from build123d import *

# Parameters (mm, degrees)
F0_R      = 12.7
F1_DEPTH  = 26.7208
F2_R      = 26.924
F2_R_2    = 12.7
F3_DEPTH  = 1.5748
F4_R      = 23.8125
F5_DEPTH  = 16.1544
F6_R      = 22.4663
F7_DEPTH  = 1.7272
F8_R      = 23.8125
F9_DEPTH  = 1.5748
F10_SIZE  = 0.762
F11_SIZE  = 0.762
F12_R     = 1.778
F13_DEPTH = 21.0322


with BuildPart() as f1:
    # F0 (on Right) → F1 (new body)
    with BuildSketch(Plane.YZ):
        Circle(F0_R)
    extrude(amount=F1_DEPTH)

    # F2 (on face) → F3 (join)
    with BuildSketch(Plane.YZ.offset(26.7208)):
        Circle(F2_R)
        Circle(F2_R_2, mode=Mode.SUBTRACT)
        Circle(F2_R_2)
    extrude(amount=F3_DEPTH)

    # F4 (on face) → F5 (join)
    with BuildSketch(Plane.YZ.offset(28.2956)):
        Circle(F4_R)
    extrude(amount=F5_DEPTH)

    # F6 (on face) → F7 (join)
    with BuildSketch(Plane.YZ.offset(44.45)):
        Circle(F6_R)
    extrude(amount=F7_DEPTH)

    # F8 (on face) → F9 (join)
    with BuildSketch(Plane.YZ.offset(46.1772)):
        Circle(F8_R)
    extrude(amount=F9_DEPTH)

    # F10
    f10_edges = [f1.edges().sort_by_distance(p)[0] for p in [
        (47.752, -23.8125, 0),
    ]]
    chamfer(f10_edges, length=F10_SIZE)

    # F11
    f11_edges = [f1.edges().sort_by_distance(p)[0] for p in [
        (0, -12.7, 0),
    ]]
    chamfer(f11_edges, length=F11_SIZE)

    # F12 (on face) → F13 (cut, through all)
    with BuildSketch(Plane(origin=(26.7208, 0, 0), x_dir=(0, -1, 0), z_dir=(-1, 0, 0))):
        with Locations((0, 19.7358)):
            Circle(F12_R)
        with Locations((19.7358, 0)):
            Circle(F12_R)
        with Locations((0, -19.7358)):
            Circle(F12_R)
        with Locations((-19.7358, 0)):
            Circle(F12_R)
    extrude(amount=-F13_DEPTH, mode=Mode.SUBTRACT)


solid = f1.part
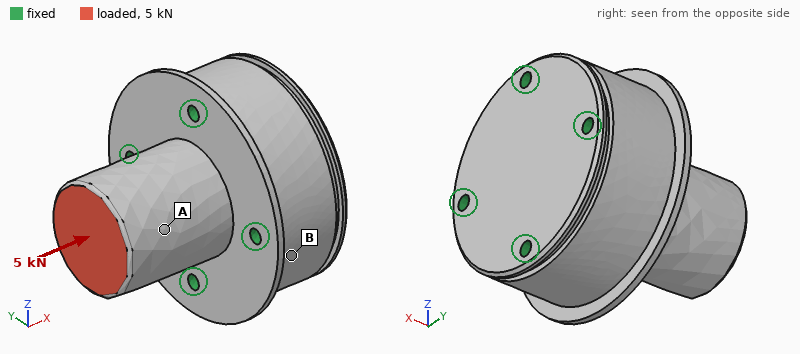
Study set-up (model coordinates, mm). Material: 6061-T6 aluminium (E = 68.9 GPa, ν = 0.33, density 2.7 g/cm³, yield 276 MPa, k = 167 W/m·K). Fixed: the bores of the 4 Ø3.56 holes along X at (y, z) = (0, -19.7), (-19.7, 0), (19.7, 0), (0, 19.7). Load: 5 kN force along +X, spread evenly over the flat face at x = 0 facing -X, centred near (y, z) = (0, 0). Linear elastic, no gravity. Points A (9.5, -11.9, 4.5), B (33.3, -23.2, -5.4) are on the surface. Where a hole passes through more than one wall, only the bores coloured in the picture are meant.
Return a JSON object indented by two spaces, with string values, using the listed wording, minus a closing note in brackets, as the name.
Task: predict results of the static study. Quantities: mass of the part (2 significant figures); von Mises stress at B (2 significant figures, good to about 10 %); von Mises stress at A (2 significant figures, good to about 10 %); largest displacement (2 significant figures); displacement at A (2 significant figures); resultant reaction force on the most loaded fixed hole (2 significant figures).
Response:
{
  "mass of the part": "140 g",
  "von Mises stress at B": "2.8 MPa",
  "von Mises stress at A": "9.2 MPa",
  "largest displacement": "6.1 µm",
  "displacement at A": "4.6 µm",
  "resultant reaction force on the most loaded fixed hole": "1.3 kN"
}
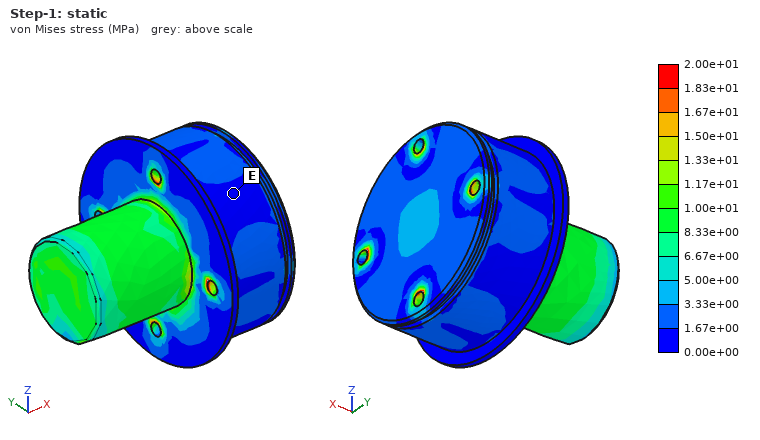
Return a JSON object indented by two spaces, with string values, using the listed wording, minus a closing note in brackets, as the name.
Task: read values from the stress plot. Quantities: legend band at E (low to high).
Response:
{
  "legend band at E": "0.00e+00 to 1.67e+00 MPa"
}
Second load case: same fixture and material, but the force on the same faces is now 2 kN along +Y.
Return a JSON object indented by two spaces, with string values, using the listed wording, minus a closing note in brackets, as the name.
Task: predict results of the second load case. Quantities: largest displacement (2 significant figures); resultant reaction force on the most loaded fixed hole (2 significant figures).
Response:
{
  "largest displacement": "23 µm",
  "resultant reaction force on the most loaded fixed hole": "1.7 kN"
}
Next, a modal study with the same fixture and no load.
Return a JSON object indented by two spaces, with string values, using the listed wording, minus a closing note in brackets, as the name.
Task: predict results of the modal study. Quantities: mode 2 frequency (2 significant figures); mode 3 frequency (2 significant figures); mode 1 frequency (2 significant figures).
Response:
{
  "mode 2 frequency": "13 kHz",
  "mode 3 frequency": "25 kHz",
  "mode 1 frequency": "13 kHz"
}
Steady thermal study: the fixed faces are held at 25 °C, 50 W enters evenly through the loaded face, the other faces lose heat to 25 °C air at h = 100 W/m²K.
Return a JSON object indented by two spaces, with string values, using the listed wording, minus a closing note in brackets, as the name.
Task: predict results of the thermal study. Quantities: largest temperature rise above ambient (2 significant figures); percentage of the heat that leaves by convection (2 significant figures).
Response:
{
  "largest temperature rise above ambient": "20 K",
  "percentage of the heat that leaves by convection": "6.4 %"
}
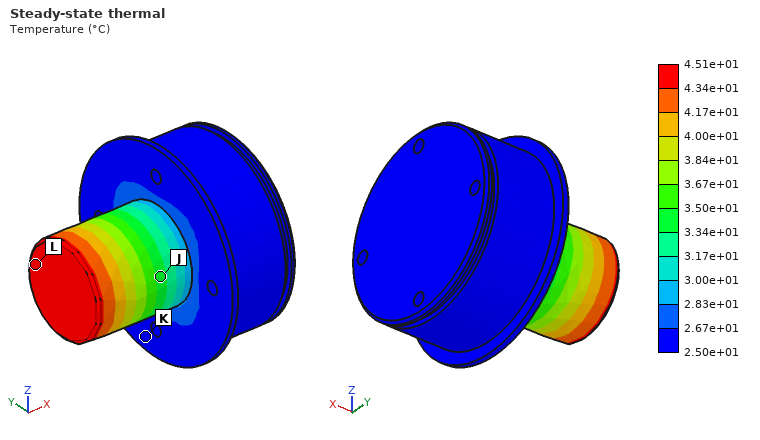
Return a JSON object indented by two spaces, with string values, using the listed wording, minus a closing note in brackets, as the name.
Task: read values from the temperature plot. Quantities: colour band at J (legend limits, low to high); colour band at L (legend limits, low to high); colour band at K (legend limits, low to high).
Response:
{
  "colour band at J": "3.34e+01 to 3.50e+01 °C",
  "colour band at L": "4.34e+01 to 4.51e+01 °C",
  "colour band at K": "2.50e+01 to 2.67e+01 °C"
}
